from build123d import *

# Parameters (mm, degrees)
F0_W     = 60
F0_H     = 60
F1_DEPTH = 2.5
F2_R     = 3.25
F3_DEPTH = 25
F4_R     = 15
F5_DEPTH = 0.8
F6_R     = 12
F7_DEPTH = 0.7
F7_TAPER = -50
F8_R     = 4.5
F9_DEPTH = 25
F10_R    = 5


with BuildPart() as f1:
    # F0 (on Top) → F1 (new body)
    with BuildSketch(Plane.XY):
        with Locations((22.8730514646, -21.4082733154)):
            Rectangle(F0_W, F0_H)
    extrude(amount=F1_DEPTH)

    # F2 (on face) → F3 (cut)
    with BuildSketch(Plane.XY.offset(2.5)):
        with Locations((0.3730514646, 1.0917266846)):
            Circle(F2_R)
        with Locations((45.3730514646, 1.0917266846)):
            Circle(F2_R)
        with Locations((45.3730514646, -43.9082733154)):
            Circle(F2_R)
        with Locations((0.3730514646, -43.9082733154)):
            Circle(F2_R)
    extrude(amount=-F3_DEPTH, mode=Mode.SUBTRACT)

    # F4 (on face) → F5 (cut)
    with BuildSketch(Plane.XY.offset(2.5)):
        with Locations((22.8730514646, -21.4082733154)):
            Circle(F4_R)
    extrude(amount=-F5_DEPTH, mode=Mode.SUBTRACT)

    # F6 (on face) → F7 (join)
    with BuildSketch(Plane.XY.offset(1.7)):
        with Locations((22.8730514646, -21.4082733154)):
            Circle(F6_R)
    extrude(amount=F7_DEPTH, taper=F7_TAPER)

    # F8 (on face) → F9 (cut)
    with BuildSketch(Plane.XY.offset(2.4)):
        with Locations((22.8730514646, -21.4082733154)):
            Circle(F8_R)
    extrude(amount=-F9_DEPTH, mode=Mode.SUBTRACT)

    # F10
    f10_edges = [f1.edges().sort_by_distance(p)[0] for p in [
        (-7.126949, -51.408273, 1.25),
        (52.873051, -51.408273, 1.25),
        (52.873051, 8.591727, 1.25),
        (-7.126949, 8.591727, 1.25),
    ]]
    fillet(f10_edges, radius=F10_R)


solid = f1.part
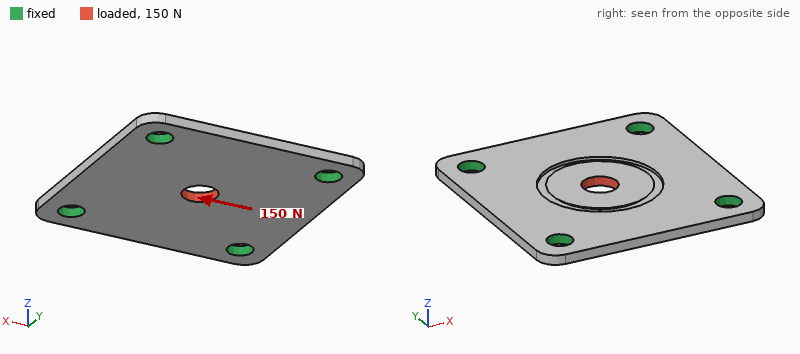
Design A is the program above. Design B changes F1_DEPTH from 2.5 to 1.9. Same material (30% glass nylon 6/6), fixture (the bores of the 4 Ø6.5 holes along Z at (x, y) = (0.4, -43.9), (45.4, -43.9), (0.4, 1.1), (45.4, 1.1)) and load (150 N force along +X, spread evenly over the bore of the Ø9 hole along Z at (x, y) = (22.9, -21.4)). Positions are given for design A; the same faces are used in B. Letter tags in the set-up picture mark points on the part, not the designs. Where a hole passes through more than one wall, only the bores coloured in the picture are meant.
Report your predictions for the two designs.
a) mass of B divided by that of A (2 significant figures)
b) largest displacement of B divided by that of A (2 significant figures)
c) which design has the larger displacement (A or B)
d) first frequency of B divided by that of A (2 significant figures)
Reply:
0.80
1.1
B
0.79
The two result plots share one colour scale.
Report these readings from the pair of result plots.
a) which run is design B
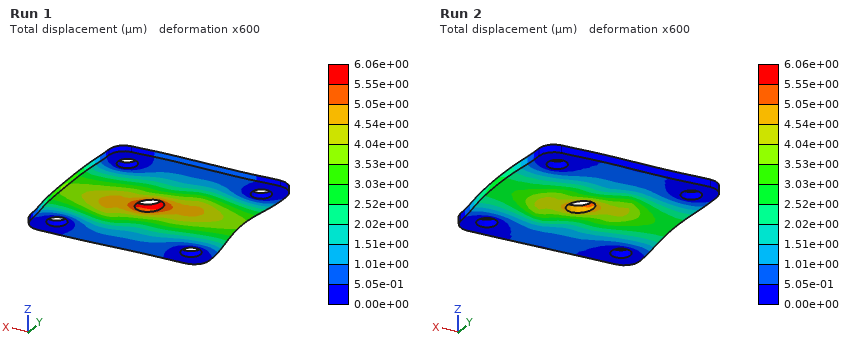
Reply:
Run 1
